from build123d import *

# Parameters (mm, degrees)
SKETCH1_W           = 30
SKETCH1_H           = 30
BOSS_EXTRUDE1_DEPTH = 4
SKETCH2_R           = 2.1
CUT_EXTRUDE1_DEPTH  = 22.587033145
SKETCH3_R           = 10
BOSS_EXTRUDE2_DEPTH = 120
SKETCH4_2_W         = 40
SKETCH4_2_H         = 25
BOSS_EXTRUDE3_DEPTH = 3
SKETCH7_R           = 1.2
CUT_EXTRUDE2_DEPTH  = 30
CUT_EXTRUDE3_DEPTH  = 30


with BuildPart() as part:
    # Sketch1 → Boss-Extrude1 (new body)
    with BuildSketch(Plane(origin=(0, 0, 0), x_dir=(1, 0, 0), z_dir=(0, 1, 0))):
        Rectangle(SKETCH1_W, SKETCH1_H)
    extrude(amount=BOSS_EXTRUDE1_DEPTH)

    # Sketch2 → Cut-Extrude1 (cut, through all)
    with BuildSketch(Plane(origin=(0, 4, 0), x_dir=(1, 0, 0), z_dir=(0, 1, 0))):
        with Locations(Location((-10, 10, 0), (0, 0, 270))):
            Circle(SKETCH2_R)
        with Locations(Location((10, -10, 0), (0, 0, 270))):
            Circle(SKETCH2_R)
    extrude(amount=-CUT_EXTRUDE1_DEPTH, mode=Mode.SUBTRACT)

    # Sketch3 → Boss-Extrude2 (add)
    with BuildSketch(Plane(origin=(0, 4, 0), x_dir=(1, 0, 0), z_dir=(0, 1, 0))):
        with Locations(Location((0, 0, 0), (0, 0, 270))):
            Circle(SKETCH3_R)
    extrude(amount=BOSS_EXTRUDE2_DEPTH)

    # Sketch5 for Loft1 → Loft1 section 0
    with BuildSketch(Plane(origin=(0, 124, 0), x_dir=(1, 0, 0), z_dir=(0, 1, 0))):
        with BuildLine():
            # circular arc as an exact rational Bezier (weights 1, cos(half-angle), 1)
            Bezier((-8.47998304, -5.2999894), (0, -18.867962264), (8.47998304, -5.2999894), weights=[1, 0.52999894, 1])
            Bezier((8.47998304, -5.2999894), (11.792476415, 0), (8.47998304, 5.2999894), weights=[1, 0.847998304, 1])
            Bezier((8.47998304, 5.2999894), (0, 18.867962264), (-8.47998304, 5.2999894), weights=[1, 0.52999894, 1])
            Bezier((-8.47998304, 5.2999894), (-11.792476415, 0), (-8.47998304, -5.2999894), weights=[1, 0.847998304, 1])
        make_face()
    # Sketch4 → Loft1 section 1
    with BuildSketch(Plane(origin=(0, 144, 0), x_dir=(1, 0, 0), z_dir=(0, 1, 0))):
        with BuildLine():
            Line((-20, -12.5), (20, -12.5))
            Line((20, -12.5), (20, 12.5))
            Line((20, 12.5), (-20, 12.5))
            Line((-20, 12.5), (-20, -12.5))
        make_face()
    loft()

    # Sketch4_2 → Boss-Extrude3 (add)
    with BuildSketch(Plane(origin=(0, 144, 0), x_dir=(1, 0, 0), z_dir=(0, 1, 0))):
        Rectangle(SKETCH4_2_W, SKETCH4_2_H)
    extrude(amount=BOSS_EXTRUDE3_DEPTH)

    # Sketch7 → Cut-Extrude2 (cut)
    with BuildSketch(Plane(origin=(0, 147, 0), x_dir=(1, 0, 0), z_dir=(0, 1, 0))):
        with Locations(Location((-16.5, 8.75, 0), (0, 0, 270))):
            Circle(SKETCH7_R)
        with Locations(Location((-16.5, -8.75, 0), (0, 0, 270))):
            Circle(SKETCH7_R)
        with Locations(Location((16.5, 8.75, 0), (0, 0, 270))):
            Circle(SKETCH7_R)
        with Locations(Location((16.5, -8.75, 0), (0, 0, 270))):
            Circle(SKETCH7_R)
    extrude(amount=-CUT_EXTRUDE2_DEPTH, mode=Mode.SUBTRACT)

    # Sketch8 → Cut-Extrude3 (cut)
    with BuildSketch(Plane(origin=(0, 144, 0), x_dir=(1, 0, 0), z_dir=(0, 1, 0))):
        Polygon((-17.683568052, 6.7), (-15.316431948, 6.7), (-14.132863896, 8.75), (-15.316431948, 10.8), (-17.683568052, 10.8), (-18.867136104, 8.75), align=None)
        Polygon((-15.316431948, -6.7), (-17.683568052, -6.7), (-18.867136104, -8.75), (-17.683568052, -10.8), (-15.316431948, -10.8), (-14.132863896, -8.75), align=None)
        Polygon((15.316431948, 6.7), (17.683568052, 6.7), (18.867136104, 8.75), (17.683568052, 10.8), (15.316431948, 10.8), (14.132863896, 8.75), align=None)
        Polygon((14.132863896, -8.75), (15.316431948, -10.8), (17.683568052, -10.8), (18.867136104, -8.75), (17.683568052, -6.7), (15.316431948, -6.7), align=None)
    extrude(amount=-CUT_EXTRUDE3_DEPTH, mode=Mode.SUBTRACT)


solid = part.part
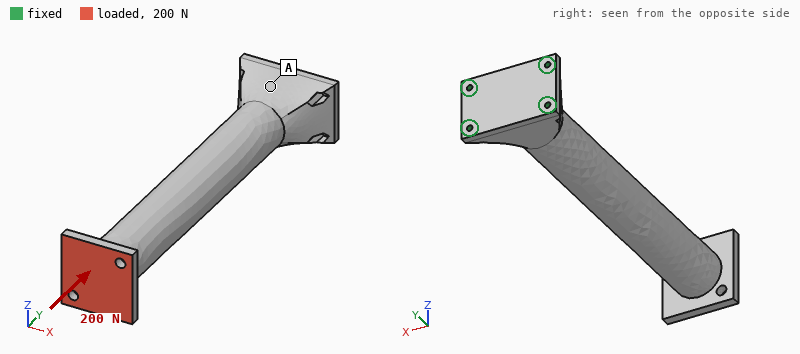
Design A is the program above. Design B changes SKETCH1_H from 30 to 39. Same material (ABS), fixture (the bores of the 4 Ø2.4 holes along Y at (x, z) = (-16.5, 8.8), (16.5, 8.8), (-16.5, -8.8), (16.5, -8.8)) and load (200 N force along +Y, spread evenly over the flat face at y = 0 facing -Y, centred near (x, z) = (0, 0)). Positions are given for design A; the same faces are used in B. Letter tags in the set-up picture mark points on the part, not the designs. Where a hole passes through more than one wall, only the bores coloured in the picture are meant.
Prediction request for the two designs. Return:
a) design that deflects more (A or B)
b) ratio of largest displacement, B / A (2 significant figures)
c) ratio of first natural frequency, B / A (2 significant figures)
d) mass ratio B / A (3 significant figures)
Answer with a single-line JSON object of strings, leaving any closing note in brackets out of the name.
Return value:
{"design that deflects more": "B", "ratio of largest displacement, B / A": "1.5", "ratio of first natural frequency, B / A": "0.96", "mass ratio B / A": "1.02"}
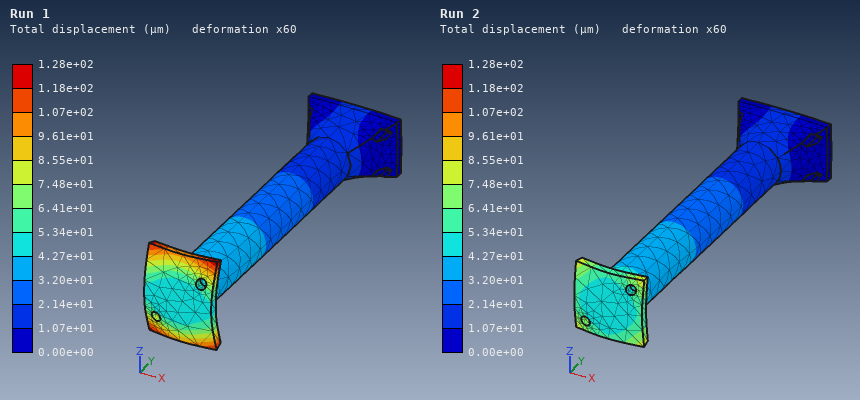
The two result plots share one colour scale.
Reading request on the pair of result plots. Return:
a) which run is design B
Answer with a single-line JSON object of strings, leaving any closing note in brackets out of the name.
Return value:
{"which run is design B": "Run 1"}
